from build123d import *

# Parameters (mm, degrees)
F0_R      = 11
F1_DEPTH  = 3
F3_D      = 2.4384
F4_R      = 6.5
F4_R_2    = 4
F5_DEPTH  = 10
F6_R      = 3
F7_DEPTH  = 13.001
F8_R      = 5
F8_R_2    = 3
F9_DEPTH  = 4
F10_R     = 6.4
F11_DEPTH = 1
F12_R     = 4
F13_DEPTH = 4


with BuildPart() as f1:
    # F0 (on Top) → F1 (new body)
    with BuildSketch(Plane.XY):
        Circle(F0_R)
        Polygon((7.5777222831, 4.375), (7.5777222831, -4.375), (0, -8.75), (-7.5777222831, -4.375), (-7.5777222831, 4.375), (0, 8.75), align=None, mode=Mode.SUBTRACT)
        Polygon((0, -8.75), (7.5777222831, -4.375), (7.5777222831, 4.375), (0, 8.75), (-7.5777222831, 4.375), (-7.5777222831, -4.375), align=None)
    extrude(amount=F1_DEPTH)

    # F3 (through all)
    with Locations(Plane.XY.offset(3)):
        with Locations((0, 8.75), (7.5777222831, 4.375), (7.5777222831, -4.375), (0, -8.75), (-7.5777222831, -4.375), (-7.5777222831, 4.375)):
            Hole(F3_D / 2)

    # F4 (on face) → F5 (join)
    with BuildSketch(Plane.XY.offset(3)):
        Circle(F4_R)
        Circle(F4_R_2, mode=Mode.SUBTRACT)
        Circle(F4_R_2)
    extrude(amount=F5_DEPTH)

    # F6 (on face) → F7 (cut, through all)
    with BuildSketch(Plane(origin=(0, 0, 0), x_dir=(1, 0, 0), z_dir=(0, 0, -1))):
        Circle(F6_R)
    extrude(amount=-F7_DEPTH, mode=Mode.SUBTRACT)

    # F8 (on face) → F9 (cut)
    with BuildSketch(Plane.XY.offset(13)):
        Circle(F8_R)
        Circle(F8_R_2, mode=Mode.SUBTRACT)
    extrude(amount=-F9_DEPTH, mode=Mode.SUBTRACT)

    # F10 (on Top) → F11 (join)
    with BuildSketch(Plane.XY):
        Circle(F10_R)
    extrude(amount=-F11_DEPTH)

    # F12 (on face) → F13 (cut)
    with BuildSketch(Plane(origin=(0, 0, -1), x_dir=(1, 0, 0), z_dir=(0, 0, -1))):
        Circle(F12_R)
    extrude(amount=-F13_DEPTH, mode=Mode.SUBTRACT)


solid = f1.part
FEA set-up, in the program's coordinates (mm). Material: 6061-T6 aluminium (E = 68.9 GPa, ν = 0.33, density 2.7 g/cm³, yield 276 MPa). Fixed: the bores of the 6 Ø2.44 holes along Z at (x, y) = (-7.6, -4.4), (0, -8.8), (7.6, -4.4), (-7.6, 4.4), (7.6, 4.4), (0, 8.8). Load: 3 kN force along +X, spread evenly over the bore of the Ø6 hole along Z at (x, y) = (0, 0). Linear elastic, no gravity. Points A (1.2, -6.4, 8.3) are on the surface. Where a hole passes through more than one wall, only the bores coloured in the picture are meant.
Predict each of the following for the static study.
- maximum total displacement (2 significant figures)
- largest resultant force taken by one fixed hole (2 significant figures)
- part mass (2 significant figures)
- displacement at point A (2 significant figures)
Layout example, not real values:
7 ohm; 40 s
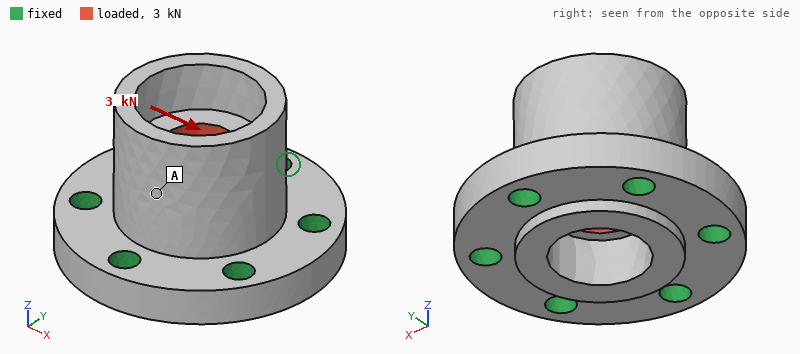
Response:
13 µm; 790 N; 4.9 g; 9.4 µm
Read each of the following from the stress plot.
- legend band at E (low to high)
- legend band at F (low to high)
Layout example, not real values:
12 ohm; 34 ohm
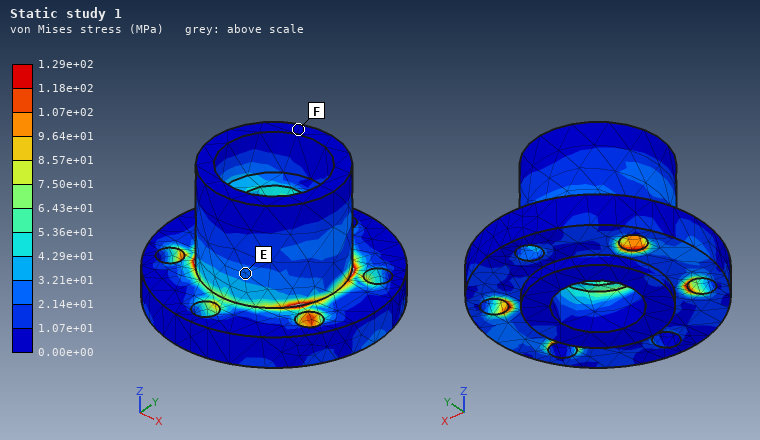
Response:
2.14e+01 to 3.21e+01 MPa; 0.00e+00 to 1.07e+01 MPa
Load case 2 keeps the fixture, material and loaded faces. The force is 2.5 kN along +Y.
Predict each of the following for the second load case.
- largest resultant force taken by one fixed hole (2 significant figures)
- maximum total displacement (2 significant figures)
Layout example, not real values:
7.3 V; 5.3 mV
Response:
750 N; 11 µm
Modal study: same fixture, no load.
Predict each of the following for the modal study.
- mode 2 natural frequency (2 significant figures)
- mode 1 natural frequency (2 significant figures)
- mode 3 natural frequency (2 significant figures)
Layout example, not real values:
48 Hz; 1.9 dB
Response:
45 kHz; 45 kHz; 59 kHz
